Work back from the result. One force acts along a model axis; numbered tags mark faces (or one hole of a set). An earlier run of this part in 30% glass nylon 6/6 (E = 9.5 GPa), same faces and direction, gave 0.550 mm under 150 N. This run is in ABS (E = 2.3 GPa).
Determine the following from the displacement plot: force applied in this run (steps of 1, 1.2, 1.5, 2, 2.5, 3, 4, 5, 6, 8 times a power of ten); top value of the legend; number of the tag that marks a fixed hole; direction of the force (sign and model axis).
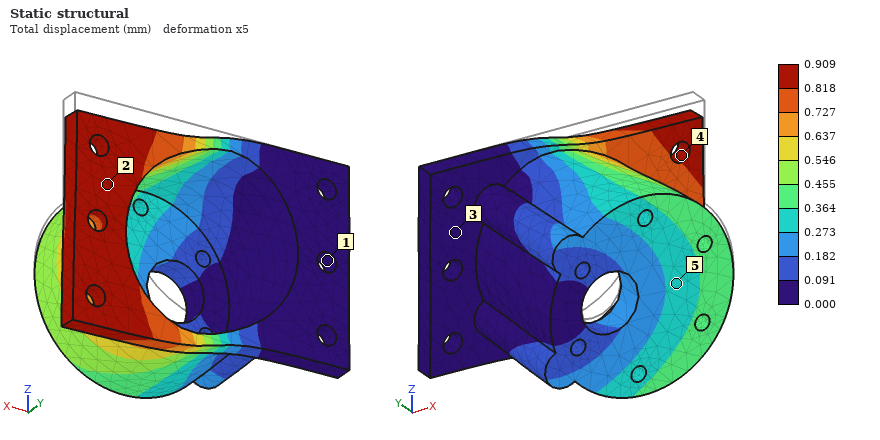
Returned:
60 N
0.909 mm
1
-Z
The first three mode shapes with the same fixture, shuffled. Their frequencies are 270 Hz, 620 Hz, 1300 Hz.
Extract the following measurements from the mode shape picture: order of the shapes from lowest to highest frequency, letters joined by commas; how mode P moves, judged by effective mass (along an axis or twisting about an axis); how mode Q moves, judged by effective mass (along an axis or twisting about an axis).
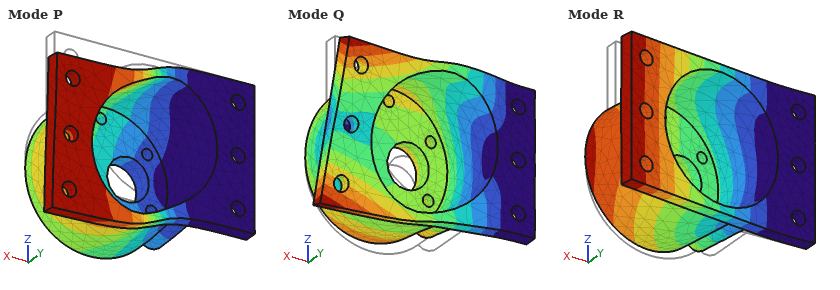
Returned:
R, P, Q
along Z
along Z
